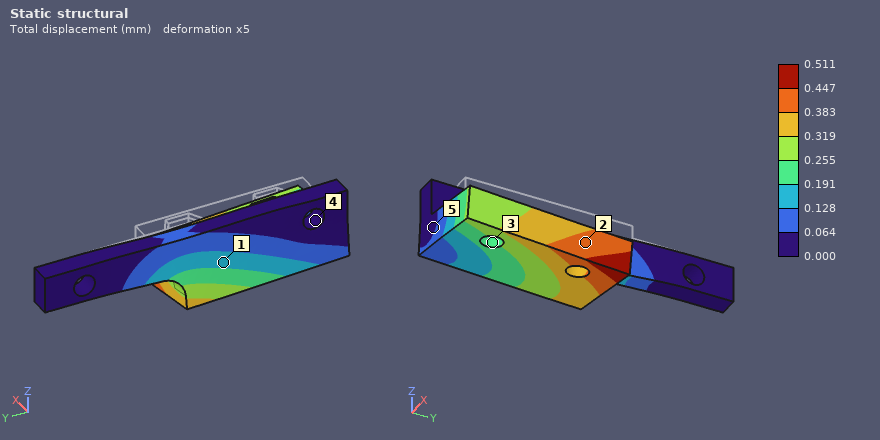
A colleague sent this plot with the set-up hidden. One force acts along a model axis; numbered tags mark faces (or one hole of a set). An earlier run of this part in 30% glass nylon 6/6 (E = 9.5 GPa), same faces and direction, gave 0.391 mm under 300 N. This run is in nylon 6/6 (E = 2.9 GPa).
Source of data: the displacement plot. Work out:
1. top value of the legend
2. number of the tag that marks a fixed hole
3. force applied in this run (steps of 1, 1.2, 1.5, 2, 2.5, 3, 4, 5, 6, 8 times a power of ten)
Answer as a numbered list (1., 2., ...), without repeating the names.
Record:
1. 0.511 mm
2. 4
3. 120 N
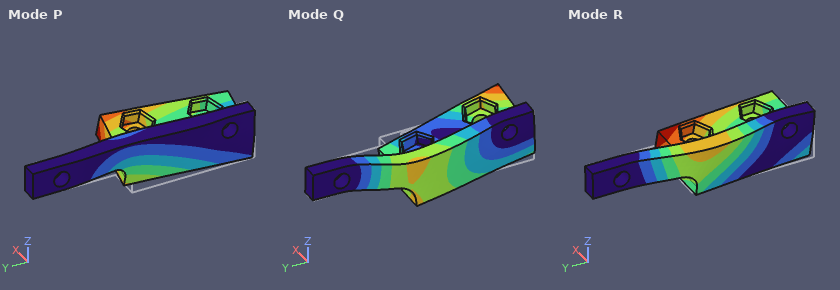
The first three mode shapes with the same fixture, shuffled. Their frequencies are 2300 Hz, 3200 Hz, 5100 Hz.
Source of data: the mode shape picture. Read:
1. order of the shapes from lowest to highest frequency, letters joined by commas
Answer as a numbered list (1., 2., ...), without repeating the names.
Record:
1. P, R, Q
